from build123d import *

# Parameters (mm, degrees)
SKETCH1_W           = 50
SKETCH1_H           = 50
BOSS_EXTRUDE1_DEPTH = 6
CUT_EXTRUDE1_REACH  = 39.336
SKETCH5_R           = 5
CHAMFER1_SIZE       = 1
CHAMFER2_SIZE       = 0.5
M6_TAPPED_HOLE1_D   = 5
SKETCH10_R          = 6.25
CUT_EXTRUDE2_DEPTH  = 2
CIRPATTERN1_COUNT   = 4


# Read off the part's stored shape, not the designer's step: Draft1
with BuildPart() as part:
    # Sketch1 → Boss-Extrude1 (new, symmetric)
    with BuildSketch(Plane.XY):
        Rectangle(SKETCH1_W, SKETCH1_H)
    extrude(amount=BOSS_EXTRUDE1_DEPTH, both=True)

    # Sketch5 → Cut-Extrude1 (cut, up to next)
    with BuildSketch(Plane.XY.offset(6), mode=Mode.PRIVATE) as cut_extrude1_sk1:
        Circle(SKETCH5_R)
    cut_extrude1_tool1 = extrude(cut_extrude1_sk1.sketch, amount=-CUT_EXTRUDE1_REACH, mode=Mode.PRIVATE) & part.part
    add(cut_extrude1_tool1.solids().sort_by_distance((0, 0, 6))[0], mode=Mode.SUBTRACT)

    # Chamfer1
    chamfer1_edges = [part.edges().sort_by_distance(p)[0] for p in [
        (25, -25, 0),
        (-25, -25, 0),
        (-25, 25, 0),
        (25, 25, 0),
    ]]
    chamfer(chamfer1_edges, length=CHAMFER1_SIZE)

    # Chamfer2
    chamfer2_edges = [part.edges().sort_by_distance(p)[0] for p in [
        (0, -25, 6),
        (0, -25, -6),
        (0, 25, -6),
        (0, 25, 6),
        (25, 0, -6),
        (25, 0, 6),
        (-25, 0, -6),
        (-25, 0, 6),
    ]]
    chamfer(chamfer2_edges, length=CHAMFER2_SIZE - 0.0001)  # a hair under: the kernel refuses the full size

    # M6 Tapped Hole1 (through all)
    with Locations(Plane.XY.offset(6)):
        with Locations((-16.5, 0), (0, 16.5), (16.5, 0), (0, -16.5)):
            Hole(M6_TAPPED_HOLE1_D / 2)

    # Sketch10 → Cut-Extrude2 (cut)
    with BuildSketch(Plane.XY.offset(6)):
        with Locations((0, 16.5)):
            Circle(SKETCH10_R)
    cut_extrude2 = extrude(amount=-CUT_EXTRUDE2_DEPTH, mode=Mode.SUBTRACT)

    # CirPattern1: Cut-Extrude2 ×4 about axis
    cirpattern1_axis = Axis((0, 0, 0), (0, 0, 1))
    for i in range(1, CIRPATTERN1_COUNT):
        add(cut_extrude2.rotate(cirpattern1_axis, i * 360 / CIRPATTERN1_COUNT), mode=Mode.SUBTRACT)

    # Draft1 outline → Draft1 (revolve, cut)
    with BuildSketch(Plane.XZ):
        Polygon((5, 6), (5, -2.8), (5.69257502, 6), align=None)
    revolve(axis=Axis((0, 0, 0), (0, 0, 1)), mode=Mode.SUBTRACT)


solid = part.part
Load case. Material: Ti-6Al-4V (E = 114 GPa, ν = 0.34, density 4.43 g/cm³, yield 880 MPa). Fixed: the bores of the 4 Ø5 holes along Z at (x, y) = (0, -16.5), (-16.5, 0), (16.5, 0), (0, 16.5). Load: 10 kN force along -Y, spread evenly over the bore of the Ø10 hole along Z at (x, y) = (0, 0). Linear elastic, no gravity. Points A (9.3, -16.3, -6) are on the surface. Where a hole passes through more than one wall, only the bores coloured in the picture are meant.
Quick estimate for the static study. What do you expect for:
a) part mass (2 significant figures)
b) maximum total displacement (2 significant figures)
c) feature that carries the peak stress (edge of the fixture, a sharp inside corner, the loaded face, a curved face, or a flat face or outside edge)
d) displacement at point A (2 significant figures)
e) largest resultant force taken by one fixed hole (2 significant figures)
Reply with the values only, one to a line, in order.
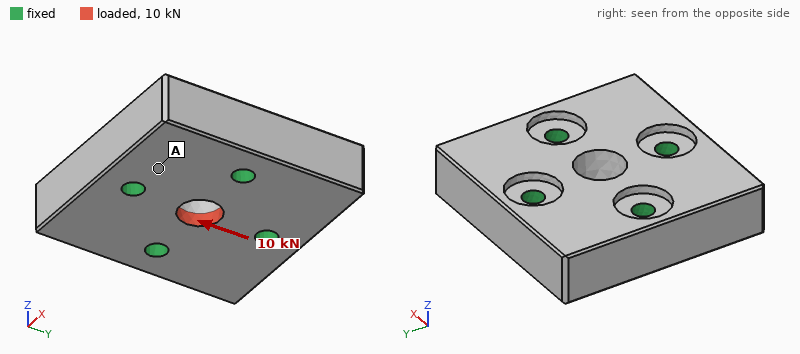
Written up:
120 g
7.1 µm
the loaded face
1.2 µm
3.4 kN
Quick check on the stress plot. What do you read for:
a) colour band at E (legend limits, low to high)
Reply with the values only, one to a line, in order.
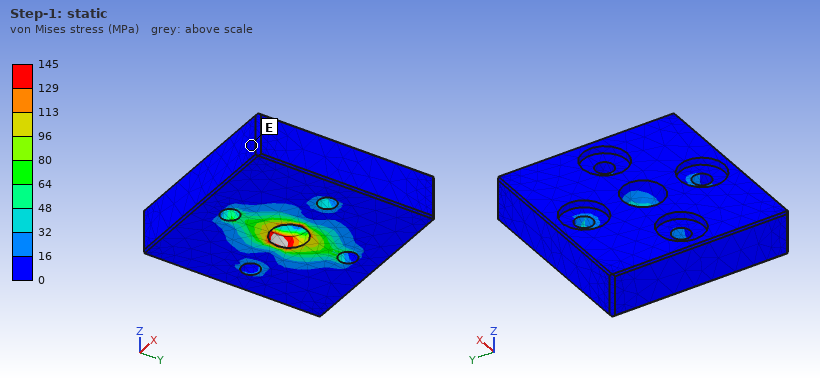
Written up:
0 to 16 MPa
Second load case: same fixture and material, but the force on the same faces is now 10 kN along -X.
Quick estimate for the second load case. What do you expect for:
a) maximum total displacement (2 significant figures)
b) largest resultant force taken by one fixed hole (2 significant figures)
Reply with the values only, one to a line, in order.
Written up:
7.0 µm
3.4 kN
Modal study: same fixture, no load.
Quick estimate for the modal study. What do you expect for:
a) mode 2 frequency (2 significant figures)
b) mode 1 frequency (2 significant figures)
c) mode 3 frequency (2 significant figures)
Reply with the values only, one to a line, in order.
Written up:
20 kHz
19 kHz
20 kHz
